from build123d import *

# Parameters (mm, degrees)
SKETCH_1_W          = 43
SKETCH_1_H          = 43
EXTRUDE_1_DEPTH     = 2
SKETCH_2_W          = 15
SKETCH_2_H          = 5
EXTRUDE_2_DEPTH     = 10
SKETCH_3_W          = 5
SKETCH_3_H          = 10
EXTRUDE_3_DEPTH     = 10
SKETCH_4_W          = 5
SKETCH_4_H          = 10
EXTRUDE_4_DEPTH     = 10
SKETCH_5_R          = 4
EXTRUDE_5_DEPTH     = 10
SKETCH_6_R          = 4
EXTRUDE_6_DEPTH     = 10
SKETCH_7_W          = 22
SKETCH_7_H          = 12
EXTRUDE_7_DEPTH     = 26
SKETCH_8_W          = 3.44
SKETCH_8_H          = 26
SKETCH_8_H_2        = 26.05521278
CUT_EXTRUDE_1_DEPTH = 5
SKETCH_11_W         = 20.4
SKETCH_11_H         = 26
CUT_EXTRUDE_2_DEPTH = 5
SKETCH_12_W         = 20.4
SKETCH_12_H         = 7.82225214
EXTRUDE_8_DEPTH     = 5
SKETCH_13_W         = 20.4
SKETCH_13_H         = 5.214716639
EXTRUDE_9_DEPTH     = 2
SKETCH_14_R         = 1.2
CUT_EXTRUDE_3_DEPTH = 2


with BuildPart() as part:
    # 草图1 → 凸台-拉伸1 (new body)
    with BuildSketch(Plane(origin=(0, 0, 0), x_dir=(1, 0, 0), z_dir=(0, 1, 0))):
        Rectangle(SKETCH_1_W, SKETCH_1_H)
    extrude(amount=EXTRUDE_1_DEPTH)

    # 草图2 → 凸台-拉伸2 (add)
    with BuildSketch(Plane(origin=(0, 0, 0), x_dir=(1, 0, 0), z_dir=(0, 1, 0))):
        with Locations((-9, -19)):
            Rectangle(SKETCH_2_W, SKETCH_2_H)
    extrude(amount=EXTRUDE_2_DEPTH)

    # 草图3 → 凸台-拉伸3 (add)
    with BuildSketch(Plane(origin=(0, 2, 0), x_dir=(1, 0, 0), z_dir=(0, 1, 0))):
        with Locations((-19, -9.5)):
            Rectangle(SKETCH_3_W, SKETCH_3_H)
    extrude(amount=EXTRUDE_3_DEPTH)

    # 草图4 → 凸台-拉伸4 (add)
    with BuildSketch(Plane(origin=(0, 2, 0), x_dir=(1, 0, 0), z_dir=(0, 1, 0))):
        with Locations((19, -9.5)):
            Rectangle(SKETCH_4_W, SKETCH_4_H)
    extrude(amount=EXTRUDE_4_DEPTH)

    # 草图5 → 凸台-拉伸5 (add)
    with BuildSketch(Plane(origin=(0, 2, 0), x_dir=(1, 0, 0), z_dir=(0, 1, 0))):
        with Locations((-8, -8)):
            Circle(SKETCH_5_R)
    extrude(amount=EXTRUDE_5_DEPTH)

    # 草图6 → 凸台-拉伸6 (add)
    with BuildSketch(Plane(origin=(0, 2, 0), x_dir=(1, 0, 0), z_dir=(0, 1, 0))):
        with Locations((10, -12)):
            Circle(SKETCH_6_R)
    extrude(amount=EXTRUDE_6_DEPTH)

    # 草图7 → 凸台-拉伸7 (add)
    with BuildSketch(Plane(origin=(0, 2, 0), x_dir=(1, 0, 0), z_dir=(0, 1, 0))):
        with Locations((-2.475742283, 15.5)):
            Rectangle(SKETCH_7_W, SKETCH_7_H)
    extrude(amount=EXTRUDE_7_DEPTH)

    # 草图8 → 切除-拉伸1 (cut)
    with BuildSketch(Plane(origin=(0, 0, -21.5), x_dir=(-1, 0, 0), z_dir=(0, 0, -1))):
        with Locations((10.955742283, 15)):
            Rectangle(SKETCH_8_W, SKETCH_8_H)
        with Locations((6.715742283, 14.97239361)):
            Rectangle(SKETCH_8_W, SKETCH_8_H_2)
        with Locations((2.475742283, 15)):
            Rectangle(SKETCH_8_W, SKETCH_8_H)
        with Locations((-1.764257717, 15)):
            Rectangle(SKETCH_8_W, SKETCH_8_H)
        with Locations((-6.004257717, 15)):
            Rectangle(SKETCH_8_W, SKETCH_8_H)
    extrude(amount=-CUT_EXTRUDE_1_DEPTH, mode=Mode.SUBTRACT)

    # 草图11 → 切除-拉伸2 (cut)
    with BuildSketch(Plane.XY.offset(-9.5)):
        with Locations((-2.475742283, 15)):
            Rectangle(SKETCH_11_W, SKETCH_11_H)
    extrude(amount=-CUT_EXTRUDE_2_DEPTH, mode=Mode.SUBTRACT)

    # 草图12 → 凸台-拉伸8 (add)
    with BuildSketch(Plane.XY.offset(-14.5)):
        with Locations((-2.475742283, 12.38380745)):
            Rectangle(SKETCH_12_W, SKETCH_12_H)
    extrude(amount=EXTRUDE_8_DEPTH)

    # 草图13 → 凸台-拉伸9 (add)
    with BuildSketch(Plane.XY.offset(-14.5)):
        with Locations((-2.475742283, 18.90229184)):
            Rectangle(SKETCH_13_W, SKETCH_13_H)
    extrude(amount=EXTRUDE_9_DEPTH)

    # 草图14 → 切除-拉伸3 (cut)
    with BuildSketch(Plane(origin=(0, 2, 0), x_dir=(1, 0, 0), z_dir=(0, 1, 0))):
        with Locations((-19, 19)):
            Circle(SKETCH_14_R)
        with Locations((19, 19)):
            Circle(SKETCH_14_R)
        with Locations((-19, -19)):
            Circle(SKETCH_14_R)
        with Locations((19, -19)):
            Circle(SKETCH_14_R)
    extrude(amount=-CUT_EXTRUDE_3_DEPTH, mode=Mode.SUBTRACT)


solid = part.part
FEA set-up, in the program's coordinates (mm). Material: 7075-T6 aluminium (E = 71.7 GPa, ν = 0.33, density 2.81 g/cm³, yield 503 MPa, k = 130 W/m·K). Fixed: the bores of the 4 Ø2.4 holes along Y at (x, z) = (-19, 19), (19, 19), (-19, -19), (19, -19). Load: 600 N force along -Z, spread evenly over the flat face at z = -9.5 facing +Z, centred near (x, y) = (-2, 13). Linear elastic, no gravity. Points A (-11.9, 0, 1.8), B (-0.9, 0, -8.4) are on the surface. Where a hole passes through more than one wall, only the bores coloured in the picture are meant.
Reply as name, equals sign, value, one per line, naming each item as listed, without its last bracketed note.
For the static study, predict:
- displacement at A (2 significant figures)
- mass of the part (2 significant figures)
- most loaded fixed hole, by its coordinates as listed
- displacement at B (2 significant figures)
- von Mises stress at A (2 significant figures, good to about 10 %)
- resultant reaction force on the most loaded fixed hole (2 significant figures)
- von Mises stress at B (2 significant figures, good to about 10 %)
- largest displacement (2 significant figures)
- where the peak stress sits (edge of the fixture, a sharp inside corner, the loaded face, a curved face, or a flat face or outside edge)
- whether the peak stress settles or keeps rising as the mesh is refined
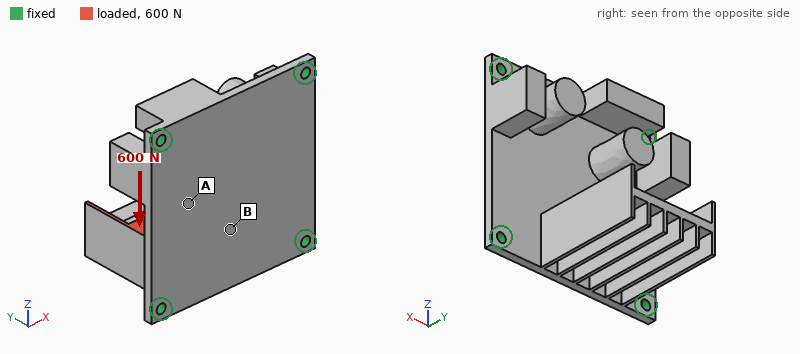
displacement at A = 0.092 mm
mass of the part = 26 g
most loaded fixed hole, by its coordinates as listed = (-19, -19)
displacement at B = 0.084 mm
von Mises stress at A = 37 MPa
resultant reaction force on the most loaded fixed hole = 260 N
von Mises stress at B = 83 MPa
largest displacement = 0.43 mm
where the peak stress sits = edge of the fixture
whether the peak stress settles or keeps rising as the mesh is refined = keeps rising
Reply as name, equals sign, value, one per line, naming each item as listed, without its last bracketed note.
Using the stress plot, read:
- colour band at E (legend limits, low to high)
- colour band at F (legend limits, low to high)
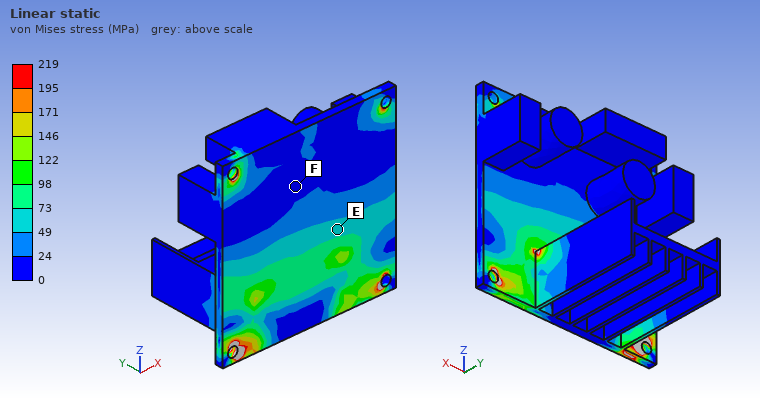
colour band at E = 49 to 73 MPa
colour band at F = 0 to 24 MPa
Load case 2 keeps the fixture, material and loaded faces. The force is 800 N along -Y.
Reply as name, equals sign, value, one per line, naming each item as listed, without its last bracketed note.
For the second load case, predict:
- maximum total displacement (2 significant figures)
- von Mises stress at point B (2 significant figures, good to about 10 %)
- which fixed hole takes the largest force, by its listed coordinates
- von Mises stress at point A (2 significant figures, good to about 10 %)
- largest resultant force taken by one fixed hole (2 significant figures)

maximum total displacement = 0.34 mm
von Mises stress at point B = 82 MPa
which fixed hole takes the largest force, by its listed coordinates = (-19, -19)
von Mises stress at point A = 36 MPa
largest resultant force taken by one fixed hole = 370 N
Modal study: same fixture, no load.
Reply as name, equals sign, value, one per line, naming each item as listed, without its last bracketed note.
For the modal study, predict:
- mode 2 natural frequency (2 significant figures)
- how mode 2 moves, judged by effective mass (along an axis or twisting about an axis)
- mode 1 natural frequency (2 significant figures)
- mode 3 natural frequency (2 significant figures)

mode 2 natural frequency = 4000 Hz
how mode 2 moves, judged by effective mass = along Y
mode 1 natural frequency = 2300 Hz
mode 3 natural frequency = 5100 Hz
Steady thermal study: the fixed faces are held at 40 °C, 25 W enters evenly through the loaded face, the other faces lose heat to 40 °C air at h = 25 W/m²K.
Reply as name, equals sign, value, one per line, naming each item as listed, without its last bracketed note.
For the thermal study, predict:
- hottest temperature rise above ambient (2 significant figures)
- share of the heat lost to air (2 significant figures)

hottest temperature rise above ambient = 53 K
share of the heat lost to air = 20 %
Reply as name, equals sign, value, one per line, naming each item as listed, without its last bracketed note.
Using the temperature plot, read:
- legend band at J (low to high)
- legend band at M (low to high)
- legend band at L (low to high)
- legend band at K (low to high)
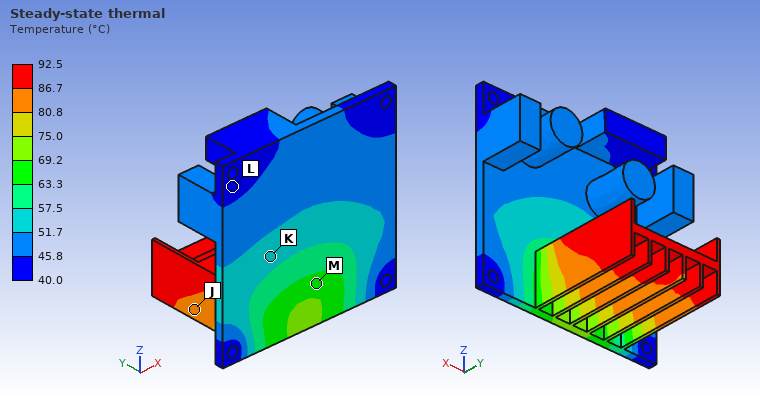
legend band at J = 80.8 to 86.7 °C
legend band at M = 63.3 to 69.2 °C
legend band at L = 40.0 to 45.8 °C
legend band at K = 51.7 to 57.5 °C
